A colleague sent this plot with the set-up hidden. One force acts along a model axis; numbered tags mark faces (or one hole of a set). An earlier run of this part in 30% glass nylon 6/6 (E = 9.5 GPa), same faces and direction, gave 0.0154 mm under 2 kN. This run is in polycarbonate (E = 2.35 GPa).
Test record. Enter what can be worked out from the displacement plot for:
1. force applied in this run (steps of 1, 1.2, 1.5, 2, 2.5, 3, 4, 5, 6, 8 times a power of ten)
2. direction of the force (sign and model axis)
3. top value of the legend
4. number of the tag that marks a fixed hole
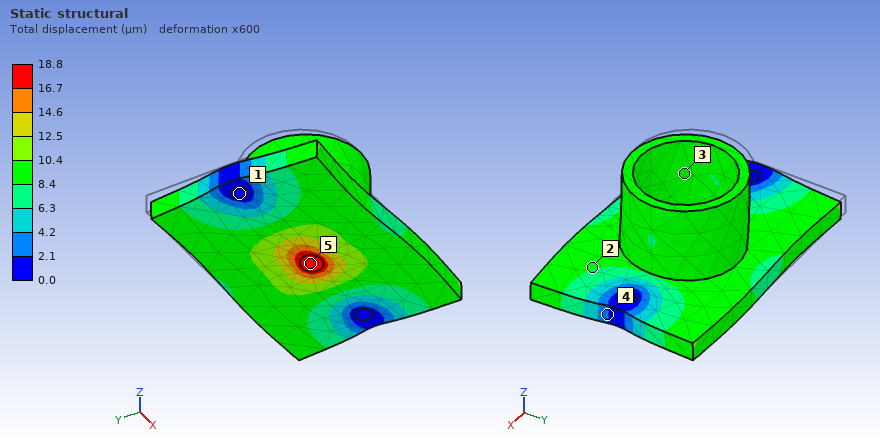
600 N
+X
18.8 µm
1
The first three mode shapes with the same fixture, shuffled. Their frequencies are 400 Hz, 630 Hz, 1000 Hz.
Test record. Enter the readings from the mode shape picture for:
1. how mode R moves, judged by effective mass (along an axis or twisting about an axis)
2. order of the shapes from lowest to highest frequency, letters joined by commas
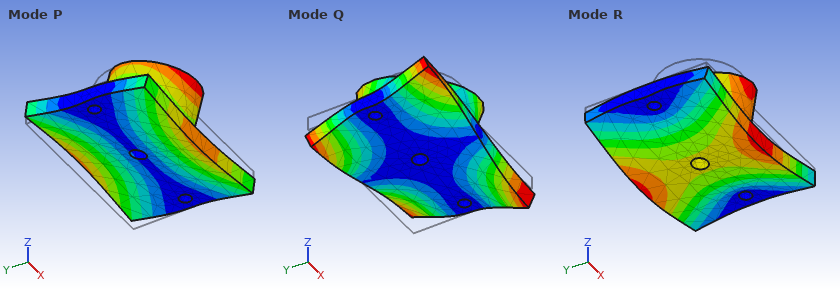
along Z
P, R, Q
